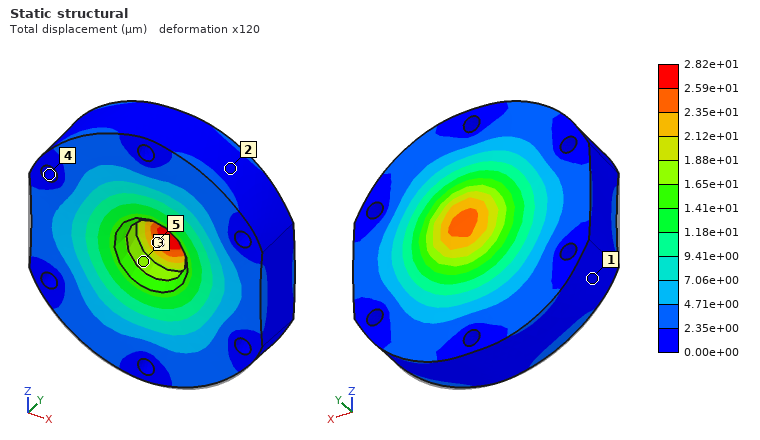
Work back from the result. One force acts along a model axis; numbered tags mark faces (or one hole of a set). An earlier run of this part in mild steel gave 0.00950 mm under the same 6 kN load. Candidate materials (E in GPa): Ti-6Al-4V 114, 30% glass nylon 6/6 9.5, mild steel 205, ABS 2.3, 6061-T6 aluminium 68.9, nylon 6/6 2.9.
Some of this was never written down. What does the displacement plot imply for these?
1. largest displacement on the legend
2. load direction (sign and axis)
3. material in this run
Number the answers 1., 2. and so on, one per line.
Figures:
1. 2.82e+01 µm
2. +Y
3. 6061-T6 aluminium
